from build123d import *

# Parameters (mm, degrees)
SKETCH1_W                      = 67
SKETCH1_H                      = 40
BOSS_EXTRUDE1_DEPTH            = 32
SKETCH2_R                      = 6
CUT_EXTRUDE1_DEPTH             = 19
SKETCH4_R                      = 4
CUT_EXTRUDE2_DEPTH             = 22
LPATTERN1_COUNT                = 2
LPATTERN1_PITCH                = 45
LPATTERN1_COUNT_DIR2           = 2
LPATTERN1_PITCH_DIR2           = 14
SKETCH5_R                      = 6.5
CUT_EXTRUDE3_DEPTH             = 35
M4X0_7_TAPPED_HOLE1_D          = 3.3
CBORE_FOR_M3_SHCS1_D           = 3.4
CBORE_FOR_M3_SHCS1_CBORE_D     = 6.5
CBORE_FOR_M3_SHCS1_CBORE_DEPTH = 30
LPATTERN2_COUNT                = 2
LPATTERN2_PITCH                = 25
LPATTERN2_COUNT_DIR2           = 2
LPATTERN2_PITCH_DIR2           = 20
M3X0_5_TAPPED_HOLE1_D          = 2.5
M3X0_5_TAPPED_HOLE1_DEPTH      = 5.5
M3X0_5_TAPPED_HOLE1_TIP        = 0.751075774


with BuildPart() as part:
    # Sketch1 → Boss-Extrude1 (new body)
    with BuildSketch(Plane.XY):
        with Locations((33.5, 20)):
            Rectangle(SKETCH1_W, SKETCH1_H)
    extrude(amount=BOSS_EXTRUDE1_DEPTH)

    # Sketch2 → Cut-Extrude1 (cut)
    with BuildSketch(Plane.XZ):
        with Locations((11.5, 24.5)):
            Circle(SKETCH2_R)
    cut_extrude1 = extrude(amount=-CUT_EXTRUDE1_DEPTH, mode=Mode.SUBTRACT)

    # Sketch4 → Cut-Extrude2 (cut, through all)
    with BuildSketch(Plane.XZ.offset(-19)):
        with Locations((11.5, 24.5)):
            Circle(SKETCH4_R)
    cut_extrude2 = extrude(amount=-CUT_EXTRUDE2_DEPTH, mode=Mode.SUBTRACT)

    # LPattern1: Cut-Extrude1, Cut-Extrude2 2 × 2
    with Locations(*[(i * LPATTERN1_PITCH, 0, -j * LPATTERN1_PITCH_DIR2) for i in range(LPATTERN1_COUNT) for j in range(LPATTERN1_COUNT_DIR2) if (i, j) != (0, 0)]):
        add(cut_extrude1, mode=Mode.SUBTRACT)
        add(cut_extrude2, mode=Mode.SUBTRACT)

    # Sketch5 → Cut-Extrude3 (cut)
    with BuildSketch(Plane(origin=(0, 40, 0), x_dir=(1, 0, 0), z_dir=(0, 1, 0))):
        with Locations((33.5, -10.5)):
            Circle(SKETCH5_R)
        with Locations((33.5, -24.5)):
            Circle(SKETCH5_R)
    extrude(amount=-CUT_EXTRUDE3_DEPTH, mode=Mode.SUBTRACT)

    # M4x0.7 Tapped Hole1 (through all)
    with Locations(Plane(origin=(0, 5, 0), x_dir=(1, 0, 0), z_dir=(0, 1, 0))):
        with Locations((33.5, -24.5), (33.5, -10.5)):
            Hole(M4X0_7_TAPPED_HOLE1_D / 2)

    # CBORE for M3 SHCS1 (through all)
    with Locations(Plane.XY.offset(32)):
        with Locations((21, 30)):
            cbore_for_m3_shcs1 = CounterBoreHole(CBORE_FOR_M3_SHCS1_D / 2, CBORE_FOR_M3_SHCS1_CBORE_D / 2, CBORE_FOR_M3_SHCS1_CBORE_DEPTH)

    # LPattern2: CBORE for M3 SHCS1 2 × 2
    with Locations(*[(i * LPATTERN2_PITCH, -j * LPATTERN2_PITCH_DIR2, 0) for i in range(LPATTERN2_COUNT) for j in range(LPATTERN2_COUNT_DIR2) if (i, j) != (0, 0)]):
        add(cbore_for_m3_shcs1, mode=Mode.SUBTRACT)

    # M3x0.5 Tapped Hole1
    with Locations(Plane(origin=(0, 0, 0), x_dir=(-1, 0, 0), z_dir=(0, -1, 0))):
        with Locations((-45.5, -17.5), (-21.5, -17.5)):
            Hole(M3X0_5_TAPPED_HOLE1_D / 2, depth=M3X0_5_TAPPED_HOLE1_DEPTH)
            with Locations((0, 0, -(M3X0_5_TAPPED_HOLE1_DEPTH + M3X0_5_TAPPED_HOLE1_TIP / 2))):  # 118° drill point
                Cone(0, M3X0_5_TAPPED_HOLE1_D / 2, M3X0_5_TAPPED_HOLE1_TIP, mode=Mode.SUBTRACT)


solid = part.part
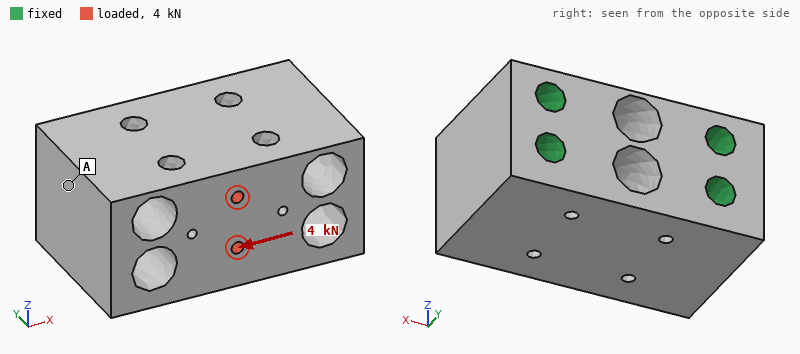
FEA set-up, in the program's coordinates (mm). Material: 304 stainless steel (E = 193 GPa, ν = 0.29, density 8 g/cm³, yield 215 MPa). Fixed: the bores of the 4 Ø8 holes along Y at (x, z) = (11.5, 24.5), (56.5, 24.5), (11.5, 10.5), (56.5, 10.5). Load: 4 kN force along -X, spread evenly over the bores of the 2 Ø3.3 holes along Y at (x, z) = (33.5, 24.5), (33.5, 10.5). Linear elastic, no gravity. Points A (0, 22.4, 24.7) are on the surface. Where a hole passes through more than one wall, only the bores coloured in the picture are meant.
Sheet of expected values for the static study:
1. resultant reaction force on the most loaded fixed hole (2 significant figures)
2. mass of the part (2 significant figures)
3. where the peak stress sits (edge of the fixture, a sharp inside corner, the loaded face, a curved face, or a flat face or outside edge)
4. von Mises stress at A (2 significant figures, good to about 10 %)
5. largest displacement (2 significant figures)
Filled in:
1.5 kN
480 g
the loaded face
5.9 MPa
3.1 µm
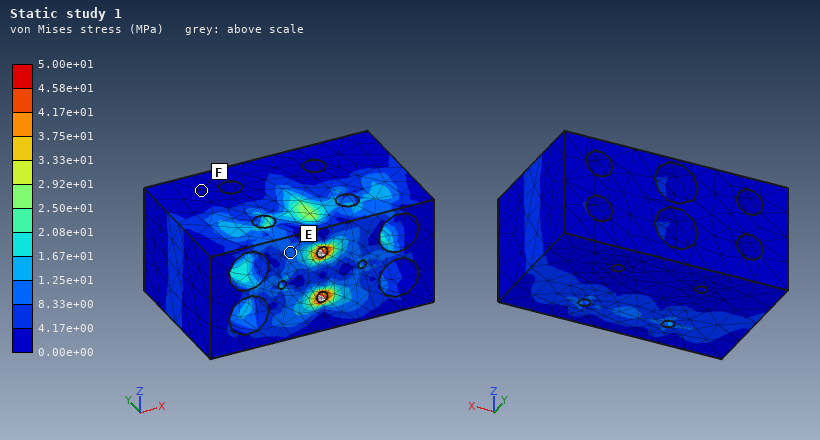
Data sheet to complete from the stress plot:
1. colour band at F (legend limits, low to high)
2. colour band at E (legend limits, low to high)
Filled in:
0.00e+00 to 4.17e+00 MPa
8.33e+00 to 1.25e+01 MPa
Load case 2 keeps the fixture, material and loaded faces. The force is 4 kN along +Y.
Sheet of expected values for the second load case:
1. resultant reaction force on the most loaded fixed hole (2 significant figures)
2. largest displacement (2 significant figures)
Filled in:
1.2 kN
5.3 µm
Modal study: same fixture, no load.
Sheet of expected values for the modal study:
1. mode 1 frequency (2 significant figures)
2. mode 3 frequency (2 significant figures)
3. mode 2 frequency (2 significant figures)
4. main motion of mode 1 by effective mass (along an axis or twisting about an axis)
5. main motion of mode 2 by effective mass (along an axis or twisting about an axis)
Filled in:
16 kHz
24 kHz
21 kHz
along Z
along X
